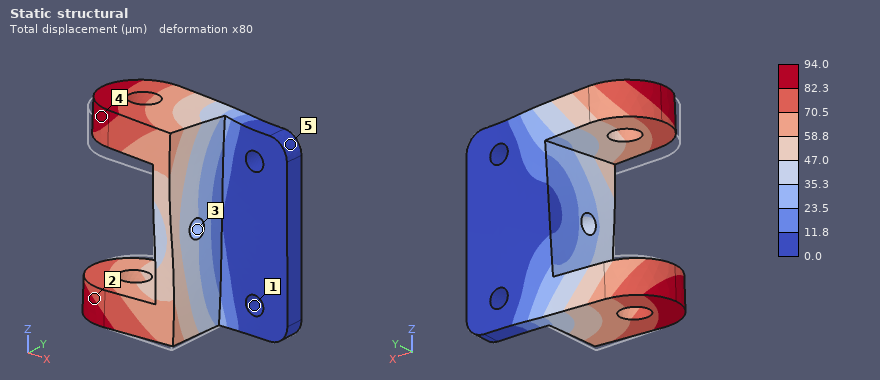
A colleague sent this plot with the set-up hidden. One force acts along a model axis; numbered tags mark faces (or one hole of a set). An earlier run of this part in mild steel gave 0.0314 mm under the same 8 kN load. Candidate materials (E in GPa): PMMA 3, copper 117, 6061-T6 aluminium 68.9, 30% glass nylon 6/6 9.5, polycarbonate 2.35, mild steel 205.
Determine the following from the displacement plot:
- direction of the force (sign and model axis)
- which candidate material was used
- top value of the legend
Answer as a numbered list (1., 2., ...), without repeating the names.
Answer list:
1. +Z
2. 6061-T6 aluminium
3. 94.0 µm
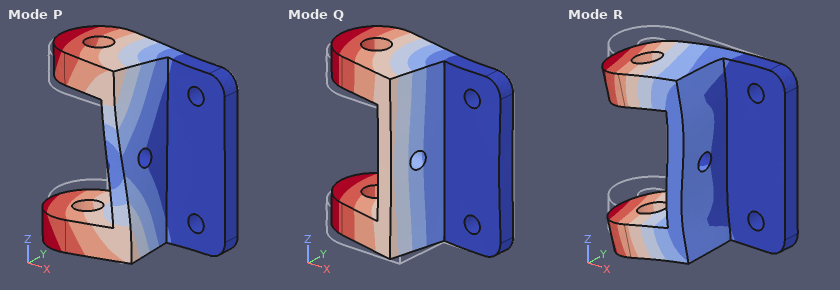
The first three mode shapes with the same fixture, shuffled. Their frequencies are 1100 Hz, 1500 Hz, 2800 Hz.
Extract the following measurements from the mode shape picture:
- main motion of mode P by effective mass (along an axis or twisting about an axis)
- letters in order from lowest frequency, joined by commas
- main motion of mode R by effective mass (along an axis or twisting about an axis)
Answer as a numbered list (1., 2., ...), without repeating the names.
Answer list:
1. twisting about X
2. Q, P, R
3. along Z
